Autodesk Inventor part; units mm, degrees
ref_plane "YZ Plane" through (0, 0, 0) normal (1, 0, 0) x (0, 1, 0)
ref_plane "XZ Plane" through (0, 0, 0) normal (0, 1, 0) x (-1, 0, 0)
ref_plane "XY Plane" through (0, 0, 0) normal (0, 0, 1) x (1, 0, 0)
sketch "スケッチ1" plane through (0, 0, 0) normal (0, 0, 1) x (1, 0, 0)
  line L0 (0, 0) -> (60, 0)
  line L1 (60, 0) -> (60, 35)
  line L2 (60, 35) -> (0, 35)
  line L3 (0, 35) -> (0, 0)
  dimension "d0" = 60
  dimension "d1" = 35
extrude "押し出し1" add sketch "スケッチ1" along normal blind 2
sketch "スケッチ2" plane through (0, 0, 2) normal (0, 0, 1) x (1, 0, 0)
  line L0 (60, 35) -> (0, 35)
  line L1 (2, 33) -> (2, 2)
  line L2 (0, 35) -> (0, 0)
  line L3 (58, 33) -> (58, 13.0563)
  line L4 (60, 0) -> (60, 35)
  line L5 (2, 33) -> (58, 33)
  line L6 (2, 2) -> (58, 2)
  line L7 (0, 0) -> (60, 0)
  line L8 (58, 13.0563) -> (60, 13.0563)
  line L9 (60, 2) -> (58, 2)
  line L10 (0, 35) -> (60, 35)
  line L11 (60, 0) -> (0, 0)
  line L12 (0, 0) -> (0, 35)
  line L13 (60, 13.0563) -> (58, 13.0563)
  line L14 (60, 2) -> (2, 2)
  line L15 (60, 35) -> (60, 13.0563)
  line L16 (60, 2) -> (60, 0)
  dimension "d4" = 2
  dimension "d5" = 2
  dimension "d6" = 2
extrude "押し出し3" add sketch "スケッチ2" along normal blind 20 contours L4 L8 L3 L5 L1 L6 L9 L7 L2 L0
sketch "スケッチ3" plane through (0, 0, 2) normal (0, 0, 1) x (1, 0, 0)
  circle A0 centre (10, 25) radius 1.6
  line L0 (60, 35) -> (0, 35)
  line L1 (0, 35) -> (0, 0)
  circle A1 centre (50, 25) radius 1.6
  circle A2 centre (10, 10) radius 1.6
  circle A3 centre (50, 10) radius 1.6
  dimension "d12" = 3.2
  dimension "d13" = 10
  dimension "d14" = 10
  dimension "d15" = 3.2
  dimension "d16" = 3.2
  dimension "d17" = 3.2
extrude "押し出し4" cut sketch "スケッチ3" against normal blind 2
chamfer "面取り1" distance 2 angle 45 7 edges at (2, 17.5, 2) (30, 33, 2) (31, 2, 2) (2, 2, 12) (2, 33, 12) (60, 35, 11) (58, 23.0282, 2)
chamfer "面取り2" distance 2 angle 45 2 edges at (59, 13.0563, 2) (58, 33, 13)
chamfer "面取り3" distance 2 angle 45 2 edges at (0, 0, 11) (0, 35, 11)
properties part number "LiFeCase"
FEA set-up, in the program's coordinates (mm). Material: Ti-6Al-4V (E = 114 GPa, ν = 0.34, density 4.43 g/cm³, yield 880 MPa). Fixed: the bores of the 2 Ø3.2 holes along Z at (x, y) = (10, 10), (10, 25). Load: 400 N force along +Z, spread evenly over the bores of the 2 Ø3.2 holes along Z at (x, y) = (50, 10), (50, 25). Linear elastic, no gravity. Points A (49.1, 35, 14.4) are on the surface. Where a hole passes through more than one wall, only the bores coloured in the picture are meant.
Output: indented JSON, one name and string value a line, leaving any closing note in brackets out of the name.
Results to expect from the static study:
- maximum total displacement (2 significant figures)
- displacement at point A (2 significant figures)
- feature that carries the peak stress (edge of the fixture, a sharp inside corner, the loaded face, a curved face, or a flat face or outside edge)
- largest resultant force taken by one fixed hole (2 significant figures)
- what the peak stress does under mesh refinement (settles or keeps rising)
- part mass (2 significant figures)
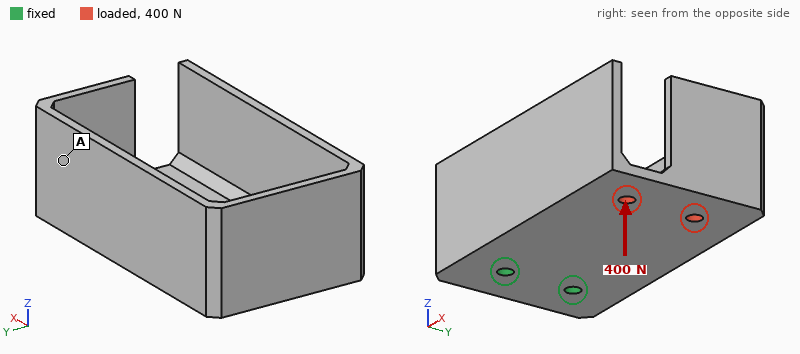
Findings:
{
  "maximum total displacement": "0.76 mm",
  "displacement at point A": "0.57 mm",
  "feature that carries the peak stress": "edge of the fixture",
  "largest resultant force taken by one fixed hole": "200 N",
  "what the peak stress does under mesh refinement": "keeps rising",
  "part mass": "50 g"
}
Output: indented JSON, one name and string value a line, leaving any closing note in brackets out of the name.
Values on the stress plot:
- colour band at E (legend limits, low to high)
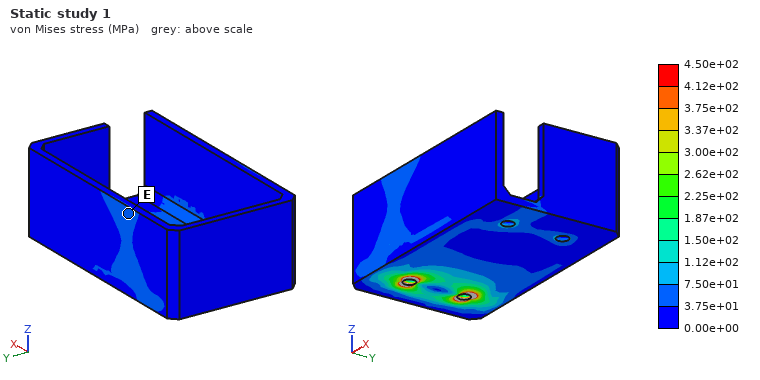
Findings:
{
  "colour band at E": "3.75e+01 to 7.50e+01 MPa"
}
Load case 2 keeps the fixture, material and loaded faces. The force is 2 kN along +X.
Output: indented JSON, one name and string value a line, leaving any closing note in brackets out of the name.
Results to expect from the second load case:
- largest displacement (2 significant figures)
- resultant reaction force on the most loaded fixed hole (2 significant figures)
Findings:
{
  "largest displacement": "16 µm",
  "resultant reaction force on the most loaded fixed hole": "1.0 kN"
}
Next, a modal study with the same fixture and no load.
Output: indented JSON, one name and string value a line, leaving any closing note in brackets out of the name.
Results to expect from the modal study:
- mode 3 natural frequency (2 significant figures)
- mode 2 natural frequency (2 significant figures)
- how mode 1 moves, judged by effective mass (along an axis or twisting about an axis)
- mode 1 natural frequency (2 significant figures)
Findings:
{
  "mode 3 natural frequency": "2900 Hz",
  "mode 2 natural frequency": "1500 Hz",
  "how mode 1 moves, judged by effective mass": "along Z",
  "mode 1 natural frequency": "830 Hz"
}
